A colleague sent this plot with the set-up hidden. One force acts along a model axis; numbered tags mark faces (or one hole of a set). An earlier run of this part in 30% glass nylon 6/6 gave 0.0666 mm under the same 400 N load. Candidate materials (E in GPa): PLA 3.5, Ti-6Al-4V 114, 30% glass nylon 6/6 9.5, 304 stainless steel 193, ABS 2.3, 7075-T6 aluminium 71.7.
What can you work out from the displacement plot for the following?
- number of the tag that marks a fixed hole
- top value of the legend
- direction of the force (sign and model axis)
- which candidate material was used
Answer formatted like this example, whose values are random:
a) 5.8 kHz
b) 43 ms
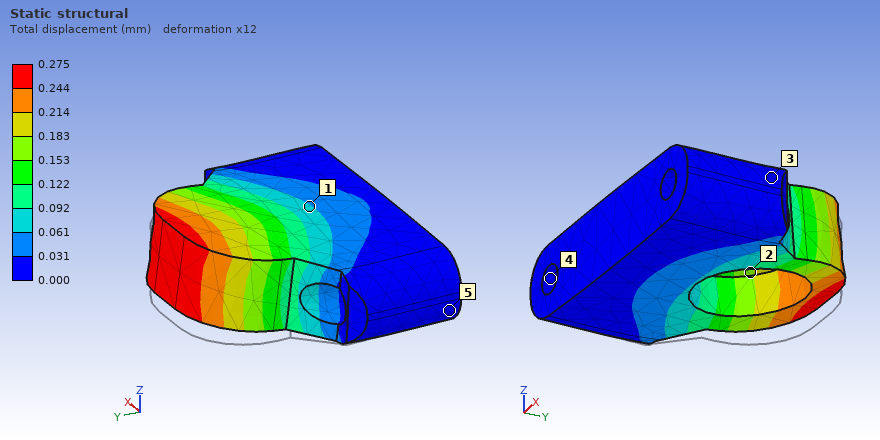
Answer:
a) 4
b) 0.275 mm
c) +Z
d) ABS
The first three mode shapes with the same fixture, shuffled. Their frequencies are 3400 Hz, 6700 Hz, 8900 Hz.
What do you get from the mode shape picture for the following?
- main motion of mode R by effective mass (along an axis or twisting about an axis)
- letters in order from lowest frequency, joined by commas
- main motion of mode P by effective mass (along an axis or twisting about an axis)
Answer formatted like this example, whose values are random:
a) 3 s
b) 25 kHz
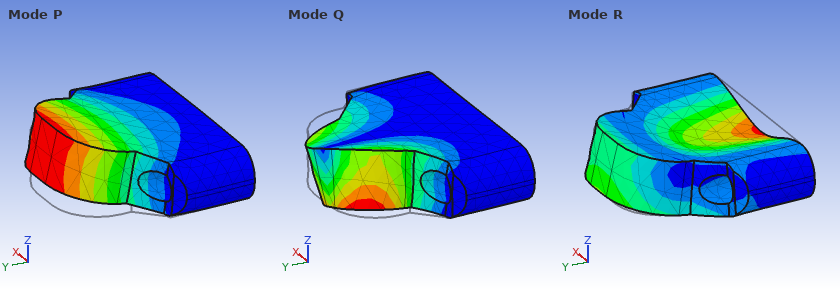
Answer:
a) along Z
b) P, Q, R
c) along Z
